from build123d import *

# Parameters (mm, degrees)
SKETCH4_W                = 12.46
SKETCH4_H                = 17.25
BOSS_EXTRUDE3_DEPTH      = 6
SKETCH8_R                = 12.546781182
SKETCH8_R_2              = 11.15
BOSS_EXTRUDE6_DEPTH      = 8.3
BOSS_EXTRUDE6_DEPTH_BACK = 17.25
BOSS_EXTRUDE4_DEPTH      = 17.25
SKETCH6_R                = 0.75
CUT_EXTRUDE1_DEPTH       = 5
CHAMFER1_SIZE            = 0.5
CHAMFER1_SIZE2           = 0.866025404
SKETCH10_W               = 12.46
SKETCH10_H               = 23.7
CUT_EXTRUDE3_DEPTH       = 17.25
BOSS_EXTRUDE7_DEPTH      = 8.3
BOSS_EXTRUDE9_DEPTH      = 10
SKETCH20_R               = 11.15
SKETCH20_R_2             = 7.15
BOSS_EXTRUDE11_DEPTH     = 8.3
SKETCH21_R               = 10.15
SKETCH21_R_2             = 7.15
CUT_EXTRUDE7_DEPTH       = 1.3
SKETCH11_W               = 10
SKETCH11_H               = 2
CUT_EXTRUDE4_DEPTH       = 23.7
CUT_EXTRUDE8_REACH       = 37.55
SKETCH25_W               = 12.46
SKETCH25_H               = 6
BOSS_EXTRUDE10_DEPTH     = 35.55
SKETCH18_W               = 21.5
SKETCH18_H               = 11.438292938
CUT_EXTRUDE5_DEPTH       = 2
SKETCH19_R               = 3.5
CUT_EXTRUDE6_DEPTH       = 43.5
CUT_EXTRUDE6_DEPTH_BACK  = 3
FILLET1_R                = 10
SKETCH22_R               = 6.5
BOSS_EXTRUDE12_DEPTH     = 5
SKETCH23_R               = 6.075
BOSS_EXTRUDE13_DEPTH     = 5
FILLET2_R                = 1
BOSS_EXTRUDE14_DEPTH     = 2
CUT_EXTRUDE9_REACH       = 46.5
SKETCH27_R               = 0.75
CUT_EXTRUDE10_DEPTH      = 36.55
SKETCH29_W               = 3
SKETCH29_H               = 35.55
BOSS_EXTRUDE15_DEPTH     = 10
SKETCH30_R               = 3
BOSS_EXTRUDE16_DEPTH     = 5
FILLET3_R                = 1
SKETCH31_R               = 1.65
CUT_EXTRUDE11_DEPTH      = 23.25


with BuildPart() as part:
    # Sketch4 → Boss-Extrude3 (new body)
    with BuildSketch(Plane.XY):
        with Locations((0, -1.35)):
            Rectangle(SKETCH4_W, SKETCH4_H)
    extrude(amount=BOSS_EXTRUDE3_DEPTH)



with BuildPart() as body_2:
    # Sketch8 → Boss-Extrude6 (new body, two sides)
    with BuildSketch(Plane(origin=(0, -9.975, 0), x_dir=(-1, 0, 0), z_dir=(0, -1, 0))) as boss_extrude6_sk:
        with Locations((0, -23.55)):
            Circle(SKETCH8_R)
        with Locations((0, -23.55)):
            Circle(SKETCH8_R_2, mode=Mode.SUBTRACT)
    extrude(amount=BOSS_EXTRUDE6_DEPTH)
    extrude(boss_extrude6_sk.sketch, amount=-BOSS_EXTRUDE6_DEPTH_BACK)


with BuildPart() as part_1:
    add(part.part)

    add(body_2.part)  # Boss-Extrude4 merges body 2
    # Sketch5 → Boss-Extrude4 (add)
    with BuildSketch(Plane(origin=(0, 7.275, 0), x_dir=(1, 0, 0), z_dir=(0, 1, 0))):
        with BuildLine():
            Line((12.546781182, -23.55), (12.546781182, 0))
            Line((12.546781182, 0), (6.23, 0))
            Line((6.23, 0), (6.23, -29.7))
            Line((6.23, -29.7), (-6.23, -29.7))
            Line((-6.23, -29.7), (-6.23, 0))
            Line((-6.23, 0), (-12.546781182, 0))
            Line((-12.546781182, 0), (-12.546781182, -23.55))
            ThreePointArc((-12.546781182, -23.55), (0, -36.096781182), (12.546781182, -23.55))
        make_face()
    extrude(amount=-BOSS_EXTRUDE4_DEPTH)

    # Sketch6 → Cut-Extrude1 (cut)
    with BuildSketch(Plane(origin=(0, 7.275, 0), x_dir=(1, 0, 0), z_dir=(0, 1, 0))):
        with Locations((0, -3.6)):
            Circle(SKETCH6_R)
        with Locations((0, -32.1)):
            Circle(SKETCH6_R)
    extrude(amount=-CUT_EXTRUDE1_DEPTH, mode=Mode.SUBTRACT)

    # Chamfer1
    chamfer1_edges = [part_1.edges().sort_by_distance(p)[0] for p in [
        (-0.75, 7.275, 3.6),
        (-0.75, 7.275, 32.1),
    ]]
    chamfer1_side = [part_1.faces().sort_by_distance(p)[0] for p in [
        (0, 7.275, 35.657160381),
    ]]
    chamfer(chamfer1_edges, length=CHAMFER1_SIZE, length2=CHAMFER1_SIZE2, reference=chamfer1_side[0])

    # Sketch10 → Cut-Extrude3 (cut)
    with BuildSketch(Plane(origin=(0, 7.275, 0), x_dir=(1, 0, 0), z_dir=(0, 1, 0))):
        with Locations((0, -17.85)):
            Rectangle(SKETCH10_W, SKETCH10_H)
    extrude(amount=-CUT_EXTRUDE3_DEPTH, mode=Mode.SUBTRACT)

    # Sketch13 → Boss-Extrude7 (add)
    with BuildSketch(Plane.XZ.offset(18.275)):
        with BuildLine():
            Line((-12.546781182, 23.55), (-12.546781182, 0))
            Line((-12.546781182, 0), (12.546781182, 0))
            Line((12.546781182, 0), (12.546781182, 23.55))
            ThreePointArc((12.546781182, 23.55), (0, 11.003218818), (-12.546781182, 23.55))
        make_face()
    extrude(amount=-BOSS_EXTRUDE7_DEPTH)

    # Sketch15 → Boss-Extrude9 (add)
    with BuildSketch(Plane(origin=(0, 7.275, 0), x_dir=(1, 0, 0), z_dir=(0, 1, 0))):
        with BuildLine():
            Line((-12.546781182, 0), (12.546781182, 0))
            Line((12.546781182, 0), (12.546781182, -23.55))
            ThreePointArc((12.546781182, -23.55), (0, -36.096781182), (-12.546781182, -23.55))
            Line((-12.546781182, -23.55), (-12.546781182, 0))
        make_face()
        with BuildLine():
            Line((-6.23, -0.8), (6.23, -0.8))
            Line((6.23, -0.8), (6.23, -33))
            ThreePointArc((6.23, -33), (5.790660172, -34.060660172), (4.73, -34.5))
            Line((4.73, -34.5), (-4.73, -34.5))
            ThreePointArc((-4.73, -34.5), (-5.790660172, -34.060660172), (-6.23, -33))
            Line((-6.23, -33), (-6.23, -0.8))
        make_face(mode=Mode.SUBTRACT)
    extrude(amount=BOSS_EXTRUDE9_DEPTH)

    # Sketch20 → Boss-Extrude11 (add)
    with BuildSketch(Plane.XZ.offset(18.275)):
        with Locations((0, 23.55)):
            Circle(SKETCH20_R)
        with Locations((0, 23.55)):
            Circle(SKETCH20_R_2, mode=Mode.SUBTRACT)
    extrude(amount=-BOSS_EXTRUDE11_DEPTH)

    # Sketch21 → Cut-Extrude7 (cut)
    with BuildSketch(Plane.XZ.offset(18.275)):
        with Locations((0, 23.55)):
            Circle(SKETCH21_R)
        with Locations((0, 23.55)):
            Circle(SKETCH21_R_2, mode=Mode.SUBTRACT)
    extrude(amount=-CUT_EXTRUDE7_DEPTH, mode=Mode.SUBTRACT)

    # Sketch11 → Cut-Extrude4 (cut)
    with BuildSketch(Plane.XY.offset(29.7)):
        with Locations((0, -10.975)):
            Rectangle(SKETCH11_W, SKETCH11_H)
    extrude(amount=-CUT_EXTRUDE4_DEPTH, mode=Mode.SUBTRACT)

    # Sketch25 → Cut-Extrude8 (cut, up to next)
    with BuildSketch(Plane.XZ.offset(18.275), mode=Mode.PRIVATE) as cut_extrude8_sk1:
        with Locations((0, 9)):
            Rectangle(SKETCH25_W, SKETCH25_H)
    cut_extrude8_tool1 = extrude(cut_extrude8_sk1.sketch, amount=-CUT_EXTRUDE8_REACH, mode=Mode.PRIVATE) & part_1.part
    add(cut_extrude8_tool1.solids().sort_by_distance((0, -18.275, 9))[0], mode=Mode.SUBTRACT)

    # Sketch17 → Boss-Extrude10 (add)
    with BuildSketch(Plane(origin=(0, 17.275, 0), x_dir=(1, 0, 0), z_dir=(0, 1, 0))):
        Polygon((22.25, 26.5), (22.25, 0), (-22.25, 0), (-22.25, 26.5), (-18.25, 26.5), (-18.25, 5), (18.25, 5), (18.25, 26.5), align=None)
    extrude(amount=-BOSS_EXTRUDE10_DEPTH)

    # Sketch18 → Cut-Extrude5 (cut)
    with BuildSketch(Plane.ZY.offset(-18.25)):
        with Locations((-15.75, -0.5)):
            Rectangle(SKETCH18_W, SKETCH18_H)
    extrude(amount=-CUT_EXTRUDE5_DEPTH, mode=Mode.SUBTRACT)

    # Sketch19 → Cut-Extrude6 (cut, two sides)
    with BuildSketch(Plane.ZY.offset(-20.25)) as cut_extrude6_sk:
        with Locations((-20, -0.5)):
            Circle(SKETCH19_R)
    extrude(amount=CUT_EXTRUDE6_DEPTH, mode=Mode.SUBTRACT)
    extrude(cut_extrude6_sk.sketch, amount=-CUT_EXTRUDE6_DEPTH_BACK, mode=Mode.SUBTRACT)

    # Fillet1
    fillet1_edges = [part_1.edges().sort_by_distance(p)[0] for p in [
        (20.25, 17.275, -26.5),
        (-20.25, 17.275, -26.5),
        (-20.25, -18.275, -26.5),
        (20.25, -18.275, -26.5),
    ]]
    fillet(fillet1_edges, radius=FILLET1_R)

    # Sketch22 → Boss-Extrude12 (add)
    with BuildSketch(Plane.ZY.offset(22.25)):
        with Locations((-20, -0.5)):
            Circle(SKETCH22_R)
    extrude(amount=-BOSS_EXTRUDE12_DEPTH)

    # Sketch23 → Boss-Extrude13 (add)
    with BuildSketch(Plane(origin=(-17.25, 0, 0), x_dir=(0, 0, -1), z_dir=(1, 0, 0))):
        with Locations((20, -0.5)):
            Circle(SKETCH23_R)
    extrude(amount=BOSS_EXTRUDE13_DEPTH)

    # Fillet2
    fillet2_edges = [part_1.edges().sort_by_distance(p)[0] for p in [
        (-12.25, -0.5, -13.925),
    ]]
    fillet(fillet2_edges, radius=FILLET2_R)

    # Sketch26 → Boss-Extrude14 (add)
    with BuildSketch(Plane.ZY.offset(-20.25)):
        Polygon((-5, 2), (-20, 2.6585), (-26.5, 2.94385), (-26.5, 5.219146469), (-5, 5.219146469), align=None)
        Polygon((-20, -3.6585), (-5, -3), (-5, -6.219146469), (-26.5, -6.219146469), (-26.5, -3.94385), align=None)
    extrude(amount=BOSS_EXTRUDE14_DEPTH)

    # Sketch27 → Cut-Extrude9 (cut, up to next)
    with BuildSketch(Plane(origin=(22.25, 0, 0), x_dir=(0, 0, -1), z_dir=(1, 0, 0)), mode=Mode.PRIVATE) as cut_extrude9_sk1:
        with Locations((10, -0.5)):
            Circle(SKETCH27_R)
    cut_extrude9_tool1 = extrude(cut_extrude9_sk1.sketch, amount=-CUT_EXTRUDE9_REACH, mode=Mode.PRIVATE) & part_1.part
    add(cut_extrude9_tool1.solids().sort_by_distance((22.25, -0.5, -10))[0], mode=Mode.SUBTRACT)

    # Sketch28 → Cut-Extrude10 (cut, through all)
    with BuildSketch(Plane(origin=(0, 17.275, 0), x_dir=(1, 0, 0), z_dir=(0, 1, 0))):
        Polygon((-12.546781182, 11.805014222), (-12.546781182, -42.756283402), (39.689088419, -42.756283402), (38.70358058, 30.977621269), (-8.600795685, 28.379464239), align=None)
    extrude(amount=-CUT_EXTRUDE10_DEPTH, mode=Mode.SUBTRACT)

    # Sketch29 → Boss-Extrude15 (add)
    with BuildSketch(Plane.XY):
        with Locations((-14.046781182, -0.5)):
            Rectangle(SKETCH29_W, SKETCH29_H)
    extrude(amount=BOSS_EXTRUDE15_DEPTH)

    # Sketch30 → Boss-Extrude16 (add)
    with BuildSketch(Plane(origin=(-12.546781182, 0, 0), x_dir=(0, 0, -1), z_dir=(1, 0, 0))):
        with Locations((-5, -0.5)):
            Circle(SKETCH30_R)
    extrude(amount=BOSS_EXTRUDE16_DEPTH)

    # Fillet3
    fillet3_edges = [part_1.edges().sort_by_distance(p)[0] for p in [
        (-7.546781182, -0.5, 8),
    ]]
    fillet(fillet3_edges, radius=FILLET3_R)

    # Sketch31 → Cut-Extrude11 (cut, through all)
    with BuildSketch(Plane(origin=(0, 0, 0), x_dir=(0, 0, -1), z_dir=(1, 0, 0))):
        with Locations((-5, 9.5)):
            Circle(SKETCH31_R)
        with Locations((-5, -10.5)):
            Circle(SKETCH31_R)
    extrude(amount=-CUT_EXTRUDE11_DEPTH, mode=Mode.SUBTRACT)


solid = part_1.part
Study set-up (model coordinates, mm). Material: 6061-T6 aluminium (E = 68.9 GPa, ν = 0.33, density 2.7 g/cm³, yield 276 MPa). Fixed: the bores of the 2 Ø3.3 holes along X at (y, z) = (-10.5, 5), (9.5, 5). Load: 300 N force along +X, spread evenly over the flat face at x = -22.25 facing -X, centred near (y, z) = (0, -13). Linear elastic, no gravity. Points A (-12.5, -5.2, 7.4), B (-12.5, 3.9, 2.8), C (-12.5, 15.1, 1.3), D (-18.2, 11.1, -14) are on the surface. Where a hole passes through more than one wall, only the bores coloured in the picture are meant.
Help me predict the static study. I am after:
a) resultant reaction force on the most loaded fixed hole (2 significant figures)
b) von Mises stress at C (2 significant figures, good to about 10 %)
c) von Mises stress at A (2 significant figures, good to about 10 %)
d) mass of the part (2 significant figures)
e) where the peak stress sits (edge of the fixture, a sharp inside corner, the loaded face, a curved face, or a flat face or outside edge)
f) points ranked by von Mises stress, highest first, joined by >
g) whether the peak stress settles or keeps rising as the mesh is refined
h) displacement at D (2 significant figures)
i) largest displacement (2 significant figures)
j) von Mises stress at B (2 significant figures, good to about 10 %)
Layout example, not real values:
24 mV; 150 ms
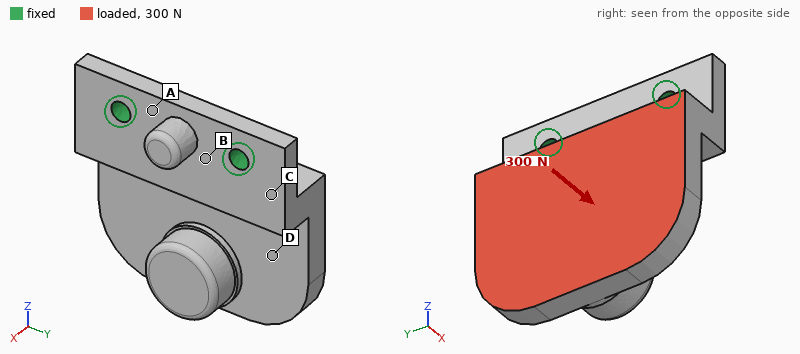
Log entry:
150 N; 64 MPa; 23 MPa; 17 g; edge of the fixture; C > B > A > D; keeps rising; 0.098 mm; 0.19 mm; 49 MPa
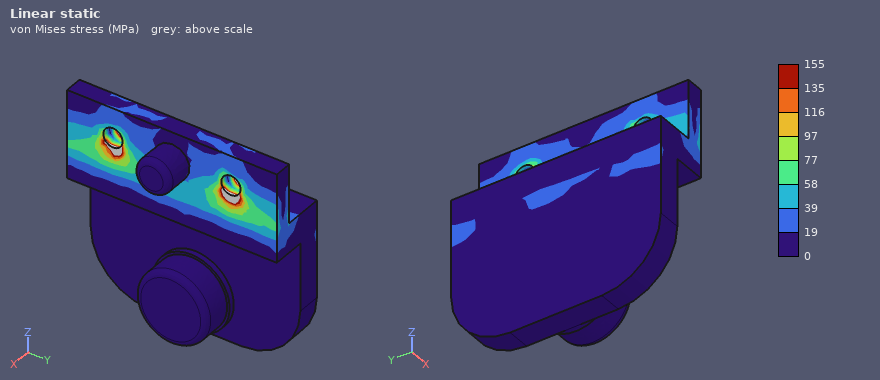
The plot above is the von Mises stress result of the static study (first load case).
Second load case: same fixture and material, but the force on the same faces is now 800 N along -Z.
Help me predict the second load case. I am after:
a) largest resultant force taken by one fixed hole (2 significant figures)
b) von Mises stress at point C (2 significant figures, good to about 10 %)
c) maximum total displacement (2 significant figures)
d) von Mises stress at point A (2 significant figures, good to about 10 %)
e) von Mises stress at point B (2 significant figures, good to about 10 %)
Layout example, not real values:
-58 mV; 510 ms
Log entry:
400 N; 96 MPa; 0.25 mm; 28 MPa; 70 MPa
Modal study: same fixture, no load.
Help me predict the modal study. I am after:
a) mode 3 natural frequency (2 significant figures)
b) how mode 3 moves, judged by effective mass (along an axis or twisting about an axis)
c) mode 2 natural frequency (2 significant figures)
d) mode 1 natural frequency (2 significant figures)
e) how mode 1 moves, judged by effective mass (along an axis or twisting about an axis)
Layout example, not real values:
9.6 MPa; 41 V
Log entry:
11 kHz; along Y; 6600 Hz; 2100 Hz; along X
